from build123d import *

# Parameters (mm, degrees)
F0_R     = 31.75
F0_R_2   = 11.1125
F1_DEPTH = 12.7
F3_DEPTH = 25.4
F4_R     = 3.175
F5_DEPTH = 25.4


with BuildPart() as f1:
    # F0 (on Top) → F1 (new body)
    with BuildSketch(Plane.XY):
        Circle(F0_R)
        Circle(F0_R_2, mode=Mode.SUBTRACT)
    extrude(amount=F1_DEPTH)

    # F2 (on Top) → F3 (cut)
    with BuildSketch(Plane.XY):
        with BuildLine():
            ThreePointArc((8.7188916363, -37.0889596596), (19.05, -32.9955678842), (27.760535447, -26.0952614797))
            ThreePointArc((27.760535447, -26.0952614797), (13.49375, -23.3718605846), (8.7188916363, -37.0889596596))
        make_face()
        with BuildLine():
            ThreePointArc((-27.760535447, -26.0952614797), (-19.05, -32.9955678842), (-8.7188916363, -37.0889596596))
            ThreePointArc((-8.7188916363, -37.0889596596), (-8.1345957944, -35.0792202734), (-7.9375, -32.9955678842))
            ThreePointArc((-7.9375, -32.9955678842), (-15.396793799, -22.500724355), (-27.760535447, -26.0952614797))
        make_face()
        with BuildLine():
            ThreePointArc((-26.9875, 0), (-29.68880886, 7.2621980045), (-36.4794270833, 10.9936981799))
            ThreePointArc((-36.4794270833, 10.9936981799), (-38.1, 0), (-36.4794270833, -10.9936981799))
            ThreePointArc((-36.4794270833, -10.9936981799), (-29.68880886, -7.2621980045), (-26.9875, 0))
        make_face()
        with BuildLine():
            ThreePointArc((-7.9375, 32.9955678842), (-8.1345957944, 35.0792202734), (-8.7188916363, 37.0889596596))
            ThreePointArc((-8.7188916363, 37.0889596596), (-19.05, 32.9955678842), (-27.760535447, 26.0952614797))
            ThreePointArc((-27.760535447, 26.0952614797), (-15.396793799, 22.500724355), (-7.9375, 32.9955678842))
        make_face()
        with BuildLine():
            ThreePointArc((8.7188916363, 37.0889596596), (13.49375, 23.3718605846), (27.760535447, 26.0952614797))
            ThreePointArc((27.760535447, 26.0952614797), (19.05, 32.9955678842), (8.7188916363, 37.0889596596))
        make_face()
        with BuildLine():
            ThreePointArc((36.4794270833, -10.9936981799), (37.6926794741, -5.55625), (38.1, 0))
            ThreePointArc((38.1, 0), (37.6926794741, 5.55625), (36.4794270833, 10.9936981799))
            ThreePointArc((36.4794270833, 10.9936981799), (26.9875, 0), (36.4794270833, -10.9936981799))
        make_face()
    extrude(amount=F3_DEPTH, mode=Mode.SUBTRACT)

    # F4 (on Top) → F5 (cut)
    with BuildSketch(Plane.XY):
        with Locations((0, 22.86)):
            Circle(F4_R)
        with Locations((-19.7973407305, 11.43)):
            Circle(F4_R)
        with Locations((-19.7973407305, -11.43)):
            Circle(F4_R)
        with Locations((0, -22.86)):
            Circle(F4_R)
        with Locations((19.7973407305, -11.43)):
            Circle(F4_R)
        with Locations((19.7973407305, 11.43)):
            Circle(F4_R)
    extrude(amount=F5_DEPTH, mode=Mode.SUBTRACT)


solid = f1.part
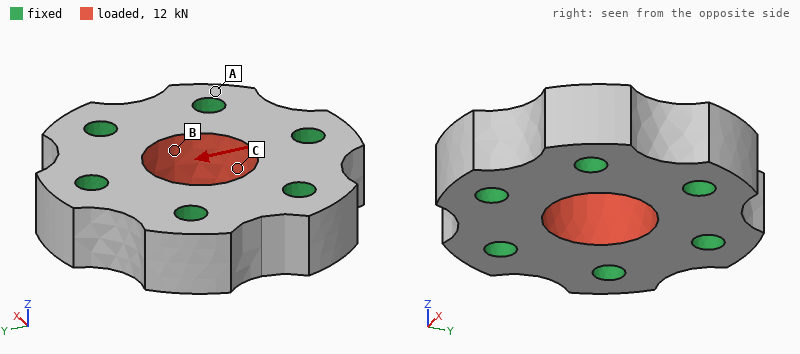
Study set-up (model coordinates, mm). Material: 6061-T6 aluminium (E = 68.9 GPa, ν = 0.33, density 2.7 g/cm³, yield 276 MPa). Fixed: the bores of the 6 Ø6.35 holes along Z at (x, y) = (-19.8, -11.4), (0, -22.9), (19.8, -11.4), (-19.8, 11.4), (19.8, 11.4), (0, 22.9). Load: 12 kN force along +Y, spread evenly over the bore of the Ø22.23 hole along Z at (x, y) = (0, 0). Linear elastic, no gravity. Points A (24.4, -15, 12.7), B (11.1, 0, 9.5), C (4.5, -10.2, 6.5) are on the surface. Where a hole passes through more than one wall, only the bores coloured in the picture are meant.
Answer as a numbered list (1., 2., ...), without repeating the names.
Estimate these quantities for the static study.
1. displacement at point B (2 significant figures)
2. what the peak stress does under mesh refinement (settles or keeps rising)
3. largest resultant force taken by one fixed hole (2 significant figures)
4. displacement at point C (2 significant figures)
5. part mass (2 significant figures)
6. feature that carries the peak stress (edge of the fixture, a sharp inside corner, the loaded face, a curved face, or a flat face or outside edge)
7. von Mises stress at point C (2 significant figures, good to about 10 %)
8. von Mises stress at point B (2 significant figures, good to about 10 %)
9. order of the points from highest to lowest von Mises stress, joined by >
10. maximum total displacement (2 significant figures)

1. 2.6 µm
2. keeps rising
3. 3.0 kN
4. 2.6 µm
5. 78 g
6. edge of the fixture
7. 14 MPa
8. 24 MPa
9. B > C > A
10. 2.9 µm
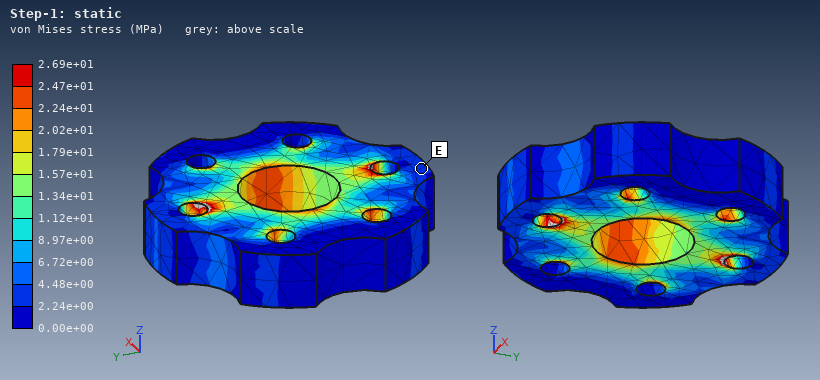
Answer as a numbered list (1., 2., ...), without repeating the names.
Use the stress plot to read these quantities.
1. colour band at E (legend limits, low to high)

1. 2.24e+00 to 4.48e+00 MPa
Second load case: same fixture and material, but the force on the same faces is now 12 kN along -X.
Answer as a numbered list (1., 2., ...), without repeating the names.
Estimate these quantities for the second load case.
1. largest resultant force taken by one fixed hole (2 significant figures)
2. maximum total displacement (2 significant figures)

1. 2.6 kN
2. 3.0 µm
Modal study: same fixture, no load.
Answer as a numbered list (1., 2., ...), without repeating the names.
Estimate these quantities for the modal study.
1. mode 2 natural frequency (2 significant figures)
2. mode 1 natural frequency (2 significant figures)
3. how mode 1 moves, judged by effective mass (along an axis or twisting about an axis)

1. 60 kHz
2. 54 kHz
3. along Z
